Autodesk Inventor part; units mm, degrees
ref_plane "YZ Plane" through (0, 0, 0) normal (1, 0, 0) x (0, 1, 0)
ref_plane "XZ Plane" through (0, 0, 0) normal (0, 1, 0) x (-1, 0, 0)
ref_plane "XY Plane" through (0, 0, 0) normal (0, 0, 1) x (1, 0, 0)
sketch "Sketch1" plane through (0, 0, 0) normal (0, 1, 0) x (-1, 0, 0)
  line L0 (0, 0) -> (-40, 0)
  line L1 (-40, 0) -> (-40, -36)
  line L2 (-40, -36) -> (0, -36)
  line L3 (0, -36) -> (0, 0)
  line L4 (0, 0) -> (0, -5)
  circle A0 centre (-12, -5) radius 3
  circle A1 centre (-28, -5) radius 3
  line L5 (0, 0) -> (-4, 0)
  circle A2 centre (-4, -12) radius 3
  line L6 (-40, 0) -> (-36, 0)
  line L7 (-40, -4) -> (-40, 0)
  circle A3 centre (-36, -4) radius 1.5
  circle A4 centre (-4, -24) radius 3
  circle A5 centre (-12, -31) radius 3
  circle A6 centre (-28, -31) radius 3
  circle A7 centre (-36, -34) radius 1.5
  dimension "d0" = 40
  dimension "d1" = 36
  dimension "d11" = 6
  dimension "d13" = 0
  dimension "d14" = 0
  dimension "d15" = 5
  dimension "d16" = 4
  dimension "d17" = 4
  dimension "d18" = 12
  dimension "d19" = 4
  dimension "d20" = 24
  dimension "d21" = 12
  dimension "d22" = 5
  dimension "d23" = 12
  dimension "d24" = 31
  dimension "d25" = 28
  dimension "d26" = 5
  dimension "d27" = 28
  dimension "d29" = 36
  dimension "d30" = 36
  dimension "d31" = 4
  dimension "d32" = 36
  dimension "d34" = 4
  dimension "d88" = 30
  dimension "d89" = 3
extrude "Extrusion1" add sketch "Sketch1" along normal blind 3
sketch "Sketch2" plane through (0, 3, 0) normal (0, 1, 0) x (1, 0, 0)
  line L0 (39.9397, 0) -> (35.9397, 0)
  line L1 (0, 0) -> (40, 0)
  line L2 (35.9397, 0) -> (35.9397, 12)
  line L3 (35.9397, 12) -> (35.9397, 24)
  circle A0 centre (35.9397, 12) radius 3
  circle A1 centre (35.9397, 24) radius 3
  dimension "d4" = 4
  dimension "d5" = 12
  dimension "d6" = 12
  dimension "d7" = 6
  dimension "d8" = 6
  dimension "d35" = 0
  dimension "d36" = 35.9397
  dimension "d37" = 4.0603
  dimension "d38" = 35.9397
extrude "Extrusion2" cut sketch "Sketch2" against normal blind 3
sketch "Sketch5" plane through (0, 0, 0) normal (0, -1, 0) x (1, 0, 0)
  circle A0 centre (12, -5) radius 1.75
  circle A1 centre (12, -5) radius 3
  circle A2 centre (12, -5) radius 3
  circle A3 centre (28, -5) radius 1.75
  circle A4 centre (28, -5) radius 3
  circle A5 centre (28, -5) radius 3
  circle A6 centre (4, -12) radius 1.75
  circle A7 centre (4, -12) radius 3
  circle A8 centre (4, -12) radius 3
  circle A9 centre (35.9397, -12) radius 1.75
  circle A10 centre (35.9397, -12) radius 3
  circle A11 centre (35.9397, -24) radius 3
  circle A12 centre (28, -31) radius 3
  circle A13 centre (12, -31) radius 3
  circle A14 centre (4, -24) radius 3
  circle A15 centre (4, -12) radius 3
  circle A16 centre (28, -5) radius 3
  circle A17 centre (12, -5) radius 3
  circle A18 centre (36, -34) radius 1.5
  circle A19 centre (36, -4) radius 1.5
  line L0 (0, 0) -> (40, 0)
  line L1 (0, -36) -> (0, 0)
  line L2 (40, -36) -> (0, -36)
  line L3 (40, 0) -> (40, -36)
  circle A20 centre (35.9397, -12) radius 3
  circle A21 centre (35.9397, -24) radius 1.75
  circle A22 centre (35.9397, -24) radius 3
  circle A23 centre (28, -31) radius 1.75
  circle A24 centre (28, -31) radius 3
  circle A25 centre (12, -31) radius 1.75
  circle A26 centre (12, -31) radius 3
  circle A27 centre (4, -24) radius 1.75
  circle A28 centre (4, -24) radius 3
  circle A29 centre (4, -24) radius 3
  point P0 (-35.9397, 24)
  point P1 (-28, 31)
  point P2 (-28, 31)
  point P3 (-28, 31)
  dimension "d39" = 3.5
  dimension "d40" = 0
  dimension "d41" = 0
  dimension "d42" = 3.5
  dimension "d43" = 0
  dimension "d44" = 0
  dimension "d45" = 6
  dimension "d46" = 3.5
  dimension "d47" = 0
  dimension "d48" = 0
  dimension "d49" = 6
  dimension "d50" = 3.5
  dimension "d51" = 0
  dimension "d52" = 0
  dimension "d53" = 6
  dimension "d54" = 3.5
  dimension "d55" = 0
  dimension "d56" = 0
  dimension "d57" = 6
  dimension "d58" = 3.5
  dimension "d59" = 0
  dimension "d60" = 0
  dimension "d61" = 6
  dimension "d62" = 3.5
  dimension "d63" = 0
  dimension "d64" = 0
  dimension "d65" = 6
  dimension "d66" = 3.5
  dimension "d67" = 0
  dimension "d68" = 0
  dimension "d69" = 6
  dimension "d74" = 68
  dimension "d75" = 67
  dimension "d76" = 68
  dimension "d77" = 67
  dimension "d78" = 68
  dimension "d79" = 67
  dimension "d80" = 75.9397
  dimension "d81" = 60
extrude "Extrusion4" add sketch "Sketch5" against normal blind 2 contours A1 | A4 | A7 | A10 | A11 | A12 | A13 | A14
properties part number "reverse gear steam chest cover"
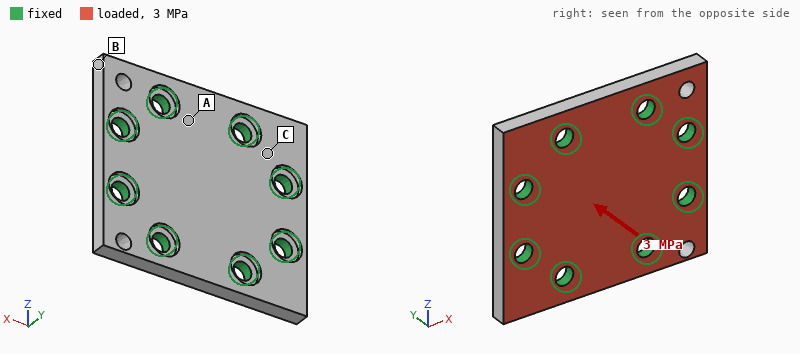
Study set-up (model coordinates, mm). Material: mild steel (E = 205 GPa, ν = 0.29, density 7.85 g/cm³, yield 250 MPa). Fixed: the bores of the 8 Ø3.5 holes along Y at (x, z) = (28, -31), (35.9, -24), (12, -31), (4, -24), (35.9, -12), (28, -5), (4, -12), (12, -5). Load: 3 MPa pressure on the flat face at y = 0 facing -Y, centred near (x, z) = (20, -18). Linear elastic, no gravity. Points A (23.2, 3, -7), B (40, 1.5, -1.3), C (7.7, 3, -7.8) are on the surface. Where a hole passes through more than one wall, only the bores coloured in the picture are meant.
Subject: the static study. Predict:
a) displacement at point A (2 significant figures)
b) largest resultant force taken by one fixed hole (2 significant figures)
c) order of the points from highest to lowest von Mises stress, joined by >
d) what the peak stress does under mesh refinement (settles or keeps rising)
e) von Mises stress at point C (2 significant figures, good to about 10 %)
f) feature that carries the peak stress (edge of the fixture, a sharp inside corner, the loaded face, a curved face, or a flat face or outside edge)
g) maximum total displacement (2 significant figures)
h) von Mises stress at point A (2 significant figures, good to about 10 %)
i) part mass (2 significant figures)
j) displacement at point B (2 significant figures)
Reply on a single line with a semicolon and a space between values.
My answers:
2.4 µm; 610 N; C > A > B; keeps rising; 54 MPa; edge of the fixture; 7.4 µm; 35 MPa; 31 g; 6.1 µm
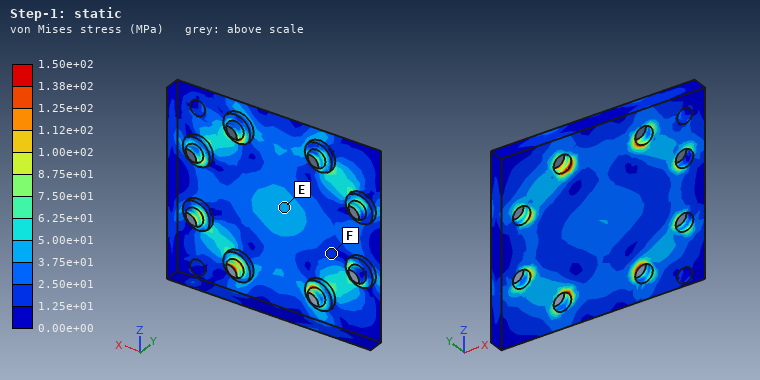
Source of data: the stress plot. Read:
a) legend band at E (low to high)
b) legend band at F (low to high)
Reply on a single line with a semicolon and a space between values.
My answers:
3.75e+01 to 5.00e+01 MPa; 1.25e+01 to 2.50e+01 MPa
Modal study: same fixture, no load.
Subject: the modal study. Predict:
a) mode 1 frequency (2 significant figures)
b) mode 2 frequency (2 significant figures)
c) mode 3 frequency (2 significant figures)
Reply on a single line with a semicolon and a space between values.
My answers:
24 kHz; 27 kHz; 27 kHz
